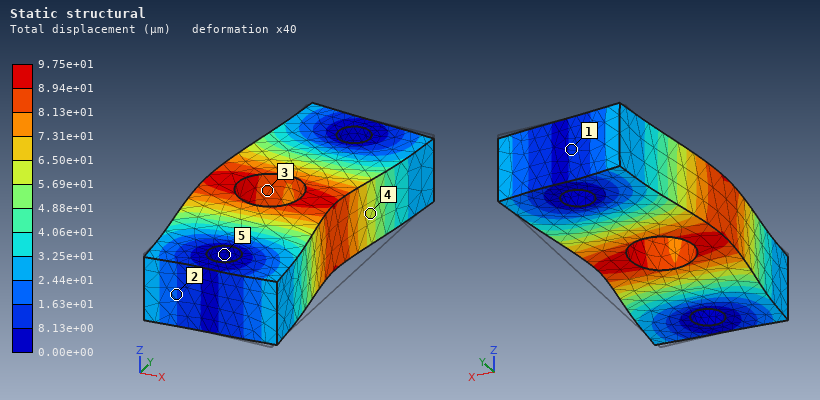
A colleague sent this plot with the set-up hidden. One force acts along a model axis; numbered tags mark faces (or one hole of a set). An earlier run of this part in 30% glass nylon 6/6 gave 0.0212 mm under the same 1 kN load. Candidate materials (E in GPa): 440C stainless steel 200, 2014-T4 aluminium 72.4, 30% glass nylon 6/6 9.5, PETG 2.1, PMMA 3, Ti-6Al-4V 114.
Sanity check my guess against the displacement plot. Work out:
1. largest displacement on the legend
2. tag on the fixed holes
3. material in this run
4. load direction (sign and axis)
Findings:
9.75e+01 µm
5
PETG
-X
